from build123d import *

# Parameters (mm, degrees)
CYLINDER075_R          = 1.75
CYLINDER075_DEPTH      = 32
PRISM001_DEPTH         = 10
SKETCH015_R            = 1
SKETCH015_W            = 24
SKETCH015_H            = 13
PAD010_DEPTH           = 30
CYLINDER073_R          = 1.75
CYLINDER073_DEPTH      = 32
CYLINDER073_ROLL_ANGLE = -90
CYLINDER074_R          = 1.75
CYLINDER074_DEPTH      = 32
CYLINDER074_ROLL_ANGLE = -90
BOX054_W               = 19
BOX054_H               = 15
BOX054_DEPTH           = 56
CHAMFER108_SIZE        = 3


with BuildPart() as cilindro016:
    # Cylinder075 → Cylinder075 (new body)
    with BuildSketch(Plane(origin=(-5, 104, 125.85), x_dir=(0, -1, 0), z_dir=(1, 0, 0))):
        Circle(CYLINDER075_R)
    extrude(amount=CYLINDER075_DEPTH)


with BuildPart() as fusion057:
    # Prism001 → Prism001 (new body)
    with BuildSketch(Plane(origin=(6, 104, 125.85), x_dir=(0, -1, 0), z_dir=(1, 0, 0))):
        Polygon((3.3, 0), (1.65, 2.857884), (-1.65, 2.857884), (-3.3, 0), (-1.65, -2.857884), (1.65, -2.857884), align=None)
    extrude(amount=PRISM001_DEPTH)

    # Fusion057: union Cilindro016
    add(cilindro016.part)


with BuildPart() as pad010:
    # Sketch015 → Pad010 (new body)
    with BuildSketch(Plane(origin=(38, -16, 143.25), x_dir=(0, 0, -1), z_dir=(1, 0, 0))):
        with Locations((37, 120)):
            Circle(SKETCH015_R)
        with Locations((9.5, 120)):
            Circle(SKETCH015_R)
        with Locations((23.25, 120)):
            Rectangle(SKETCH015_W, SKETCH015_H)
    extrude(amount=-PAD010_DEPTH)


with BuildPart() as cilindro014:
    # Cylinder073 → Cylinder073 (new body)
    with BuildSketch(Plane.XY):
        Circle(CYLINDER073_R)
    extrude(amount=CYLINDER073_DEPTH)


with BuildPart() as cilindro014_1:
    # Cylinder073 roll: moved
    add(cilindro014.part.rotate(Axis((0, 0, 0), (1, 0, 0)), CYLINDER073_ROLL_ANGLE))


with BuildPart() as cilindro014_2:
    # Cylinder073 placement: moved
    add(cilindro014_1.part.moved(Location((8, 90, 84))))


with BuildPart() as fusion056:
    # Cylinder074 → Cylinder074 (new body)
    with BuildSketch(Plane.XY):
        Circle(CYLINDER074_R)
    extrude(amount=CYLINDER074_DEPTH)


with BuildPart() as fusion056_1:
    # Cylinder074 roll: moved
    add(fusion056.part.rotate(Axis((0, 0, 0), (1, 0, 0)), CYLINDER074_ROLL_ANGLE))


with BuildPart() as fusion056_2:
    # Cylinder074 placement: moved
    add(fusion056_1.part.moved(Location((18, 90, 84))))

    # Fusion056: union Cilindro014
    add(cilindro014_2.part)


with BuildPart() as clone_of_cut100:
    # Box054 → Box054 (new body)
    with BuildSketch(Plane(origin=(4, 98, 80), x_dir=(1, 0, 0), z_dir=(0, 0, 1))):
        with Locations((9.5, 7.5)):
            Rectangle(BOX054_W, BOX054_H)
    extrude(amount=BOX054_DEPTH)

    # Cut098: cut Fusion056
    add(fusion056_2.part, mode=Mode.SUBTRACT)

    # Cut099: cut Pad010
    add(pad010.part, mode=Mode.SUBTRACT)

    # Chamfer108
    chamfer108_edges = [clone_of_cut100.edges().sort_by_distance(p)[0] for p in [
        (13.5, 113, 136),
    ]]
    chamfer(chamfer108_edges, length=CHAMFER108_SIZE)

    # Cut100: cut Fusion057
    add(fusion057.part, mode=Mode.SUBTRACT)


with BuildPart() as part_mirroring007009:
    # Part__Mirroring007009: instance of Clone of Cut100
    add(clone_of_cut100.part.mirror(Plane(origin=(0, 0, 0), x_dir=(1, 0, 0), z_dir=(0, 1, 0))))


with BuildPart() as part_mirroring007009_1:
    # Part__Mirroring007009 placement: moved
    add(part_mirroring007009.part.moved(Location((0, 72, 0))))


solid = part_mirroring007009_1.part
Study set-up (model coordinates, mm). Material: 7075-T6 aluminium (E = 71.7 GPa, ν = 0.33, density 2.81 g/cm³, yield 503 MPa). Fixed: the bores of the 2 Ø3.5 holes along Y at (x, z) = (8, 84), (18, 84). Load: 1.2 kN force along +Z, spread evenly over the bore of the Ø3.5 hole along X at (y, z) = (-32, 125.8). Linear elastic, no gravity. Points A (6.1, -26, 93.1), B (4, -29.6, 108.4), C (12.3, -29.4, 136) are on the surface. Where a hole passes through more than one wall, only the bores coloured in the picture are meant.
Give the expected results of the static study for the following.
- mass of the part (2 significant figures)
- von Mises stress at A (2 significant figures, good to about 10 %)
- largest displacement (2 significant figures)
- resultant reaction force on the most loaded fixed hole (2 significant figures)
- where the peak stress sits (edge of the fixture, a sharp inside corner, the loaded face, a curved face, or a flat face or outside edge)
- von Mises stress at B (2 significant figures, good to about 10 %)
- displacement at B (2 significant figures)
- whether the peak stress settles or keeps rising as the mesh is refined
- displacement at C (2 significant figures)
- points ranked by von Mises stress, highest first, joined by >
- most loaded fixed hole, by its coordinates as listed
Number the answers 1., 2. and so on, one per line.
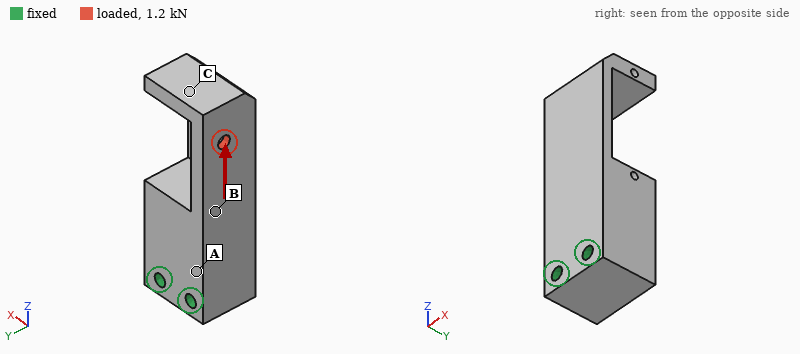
1. 31 g
2. 16 MPa
3. 42 µm
4. 1.4 kN
5. a sharp inside corner
6. 27 MPa
7. 9.4 µm
8. keeps rising
9. 36 µm
10. B > A > C
11. (8, 84)
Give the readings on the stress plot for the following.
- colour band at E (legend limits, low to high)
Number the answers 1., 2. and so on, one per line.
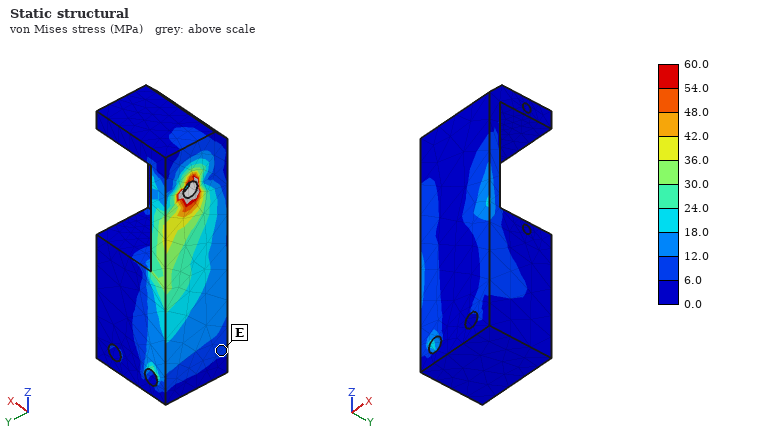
1. 6.0 to 12.0 MPa
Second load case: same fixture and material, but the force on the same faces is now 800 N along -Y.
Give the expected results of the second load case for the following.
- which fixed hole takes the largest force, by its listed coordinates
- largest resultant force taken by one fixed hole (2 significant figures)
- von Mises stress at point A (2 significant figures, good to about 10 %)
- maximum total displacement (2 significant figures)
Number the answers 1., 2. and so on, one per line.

1. (8, 84)
2. 650 N
3. 45 MPa
4. 0.14 mm
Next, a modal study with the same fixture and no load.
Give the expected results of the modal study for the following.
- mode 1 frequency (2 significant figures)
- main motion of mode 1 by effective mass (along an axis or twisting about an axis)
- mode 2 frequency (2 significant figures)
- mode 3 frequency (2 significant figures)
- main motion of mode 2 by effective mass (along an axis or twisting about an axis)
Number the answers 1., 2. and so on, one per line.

1. 4000 Hz
2. along Y
3. 4800 Hz
4. 9000 Hz
5. along X
